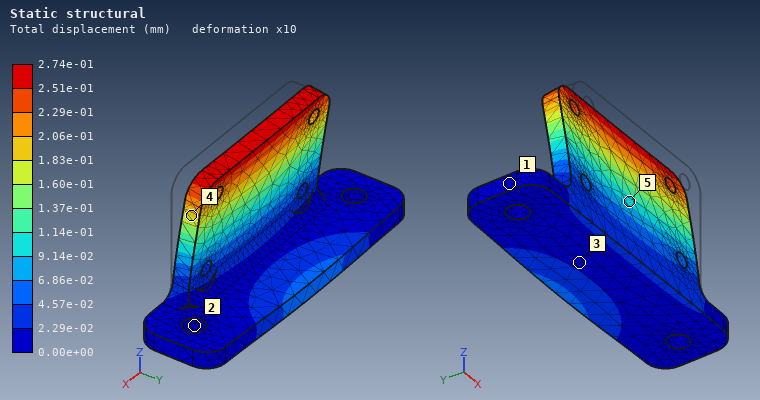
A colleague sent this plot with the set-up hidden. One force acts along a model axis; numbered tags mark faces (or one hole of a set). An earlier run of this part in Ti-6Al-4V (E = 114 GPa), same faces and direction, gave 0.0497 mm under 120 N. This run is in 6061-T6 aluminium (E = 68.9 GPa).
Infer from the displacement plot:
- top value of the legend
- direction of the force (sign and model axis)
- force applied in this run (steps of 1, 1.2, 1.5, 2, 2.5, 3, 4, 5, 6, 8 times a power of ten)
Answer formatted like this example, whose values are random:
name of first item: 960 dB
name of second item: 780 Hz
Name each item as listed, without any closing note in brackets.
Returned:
top value of the legend: 2.74e-01 mm
direction of the force: +Y
force applied in this run: 400 N
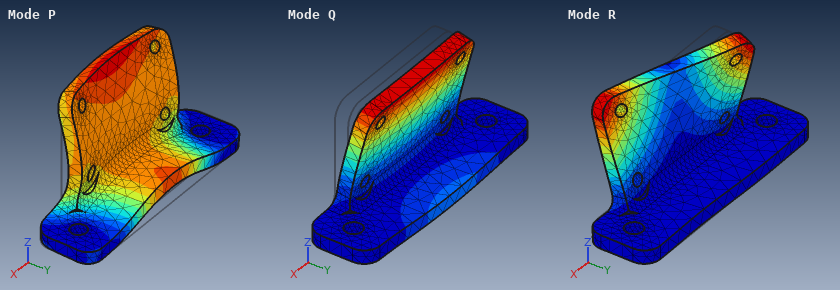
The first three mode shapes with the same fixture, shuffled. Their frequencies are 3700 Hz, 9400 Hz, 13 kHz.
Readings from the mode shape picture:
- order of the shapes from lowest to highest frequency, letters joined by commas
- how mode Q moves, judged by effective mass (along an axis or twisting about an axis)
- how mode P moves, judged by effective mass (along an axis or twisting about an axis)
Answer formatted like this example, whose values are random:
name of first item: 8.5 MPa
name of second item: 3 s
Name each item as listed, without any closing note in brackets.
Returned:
order of the shapes from lowest to highest frequency, letters joined by commas: Q, R, P
how mode Q moves, judged by effective mass: along Y
how mode P moves, judged by effective mass: along Z
